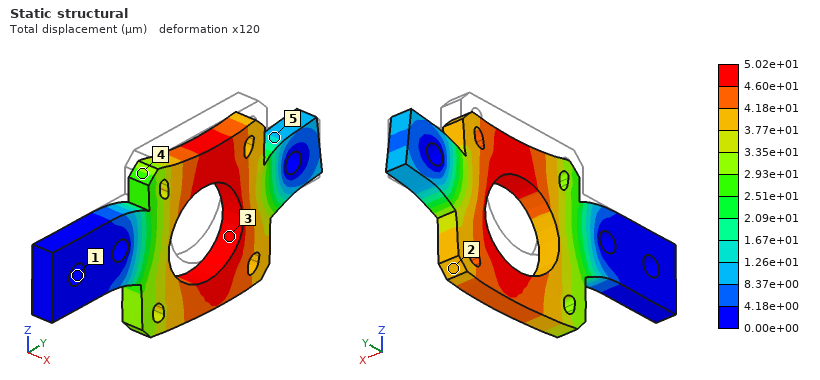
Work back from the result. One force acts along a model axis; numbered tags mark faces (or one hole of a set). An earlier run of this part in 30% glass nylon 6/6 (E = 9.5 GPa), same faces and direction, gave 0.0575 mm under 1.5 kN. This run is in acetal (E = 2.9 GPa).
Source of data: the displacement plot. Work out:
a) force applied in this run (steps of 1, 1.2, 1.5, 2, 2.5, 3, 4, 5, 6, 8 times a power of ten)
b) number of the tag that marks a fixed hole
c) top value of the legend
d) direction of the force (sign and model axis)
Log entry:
400 N
1
5.02e+01 µm
-Z
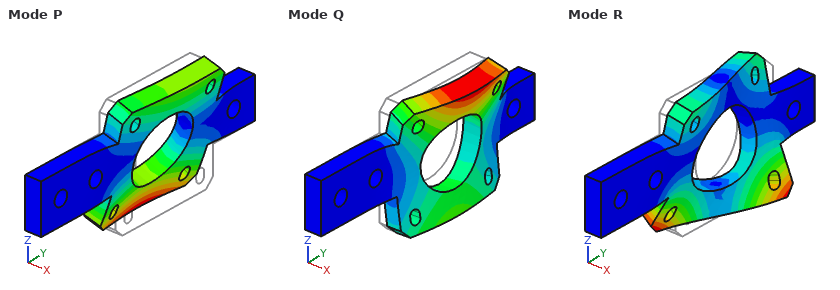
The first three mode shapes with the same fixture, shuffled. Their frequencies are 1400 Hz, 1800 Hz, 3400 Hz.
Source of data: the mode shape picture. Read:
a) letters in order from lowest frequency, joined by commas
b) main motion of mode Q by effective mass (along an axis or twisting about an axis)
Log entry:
P, Q, R
along X
